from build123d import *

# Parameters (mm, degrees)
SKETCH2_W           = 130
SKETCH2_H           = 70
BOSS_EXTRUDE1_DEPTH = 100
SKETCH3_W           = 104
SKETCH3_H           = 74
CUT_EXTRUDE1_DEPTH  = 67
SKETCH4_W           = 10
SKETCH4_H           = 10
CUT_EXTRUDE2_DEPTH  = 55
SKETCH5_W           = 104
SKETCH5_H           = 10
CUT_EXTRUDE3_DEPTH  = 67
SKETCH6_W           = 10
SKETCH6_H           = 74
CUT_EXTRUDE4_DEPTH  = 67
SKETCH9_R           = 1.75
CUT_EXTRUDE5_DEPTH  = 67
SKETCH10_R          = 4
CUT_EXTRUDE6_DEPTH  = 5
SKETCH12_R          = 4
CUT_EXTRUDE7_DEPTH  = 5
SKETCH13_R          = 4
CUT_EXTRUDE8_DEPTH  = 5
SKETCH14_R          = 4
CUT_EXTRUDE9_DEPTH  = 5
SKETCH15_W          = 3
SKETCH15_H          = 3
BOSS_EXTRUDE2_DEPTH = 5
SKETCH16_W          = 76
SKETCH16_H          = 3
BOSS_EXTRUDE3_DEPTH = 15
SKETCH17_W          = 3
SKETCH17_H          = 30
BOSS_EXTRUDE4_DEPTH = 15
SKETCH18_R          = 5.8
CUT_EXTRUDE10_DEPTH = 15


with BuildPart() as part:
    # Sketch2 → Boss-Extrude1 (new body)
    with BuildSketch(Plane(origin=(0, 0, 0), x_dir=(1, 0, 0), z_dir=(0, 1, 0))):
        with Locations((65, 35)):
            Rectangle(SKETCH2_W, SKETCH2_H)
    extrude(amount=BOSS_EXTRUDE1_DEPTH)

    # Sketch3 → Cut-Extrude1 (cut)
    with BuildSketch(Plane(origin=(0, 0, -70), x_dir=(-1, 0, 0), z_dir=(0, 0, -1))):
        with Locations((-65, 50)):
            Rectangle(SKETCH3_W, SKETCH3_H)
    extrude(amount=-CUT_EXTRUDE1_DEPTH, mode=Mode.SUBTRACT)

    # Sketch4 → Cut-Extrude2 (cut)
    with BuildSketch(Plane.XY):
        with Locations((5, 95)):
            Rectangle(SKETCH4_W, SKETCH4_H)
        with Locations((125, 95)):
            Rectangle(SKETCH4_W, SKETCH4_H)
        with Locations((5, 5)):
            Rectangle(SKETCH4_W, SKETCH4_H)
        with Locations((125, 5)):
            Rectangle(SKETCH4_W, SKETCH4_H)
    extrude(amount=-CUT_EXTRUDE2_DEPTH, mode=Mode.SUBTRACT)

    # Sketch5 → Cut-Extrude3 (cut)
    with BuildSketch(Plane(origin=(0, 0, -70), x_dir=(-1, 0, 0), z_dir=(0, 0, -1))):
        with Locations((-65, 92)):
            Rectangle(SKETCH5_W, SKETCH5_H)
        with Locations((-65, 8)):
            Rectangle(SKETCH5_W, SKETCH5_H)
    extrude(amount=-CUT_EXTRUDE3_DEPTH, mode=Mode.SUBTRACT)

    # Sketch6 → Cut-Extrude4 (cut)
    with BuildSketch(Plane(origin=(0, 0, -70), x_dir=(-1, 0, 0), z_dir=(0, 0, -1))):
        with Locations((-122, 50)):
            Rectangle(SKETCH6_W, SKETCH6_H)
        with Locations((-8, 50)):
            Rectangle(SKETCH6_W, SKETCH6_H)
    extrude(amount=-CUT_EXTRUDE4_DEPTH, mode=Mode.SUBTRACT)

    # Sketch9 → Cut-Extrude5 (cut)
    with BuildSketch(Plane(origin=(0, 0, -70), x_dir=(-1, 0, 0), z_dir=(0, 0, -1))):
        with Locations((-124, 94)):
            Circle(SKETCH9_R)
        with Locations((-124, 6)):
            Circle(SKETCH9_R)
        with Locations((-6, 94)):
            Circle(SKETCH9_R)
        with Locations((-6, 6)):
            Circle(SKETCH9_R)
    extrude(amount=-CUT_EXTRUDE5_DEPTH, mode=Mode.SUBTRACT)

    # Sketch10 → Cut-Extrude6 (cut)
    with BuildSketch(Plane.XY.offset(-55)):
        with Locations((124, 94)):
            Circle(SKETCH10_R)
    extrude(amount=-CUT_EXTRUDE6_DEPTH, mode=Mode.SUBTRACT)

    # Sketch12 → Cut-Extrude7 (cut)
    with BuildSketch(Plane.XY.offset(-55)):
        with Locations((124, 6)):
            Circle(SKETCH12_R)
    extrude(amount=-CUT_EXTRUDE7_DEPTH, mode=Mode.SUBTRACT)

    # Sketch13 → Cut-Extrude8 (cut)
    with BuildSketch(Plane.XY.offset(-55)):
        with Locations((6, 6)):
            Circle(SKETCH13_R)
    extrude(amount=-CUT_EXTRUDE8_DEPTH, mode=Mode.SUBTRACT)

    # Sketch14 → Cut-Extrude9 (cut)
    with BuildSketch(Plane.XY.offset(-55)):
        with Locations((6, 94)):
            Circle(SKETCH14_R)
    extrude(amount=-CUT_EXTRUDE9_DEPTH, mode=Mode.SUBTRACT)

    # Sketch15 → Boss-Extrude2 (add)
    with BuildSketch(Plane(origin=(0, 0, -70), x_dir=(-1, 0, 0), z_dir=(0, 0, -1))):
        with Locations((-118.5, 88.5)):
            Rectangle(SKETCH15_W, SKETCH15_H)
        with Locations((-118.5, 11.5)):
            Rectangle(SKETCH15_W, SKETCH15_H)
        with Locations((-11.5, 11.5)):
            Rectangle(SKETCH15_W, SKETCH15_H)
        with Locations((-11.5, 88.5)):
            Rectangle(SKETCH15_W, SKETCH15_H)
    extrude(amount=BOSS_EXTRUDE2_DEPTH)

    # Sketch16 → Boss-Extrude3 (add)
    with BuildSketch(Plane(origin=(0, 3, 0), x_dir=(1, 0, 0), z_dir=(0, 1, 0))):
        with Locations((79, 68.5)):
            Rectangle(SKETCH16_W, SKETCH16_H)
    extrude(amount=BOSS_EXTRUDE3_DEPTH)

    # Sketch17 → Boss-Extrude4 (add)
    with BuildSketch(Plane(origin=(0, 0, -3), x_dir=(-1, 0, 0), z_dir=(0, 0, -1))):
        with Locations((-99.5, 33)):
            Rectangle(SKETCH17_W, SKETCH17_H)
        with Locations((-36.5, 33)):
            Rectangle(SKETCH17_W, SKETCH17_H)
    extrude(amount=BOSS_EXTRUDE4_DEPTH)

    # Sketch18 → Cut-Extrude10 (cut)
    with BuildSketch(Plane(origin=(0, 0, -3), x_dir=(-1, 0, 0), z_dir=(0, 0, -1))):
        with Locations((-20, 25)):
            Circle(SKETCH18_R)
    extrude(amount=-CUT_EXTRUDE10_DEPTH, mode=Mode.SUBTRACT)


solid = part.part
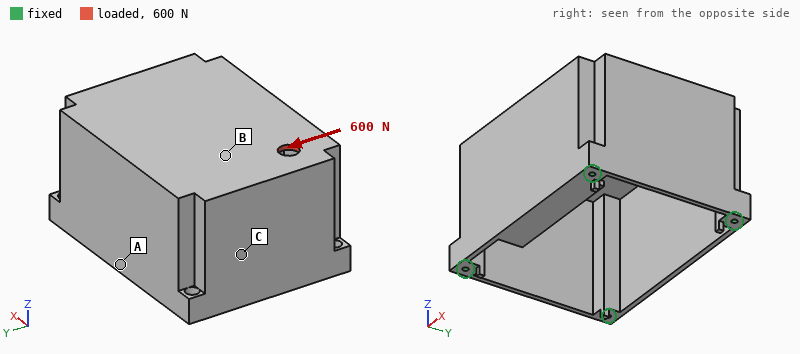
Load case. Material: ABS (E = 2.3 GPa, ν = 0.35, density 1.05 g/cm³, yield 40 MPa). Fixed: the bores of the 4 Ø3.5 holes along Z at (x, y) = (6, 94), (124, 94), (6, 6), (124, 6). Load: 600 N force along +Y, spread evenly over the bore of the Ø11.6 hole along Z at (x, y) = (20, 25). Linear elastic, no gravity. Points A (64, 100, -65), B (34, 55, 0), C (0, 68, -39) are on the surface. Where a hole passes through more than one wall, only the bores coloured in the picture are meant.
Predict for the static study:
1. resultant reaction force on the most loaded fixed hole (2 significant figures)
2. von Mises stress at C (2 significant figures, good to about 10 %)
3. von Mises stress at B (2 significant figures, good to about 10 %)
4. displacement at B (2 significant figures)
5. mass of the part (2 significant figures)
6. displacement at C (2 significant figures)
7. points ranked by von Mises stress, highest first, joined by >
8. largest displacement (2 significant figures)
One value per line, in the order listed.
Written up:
330 N
3.2 MPa
1.7 MPa
0.20 mm
150 g
0.083 mm
C > B > A
0.26 mm
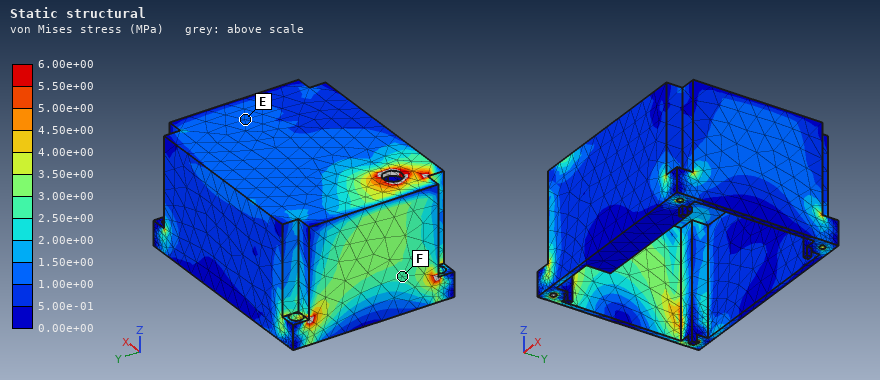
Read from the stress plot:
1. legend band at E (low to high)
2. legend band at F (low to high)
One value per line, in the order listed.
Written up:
1.00e+00 to 1.50e+00 MPa
2.50e+00 to 3.00e+00 MPa
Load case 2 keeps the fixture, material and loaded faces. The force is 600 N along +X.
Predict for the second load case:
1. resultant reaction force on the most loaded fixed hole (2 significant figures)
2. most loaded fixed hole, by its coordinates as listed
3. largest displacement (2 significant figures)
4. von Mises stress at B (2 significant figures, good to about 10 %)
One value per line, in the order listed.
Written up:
270 N
(124, 6)
0.22 mm
1.8 MPa
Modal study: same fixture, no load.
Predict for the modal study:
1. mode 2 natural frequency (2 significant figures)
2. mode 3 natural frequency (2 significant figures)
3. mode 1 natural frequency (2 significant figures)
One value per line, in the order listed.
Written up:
530 Hz
640 Hz
450 Hz
